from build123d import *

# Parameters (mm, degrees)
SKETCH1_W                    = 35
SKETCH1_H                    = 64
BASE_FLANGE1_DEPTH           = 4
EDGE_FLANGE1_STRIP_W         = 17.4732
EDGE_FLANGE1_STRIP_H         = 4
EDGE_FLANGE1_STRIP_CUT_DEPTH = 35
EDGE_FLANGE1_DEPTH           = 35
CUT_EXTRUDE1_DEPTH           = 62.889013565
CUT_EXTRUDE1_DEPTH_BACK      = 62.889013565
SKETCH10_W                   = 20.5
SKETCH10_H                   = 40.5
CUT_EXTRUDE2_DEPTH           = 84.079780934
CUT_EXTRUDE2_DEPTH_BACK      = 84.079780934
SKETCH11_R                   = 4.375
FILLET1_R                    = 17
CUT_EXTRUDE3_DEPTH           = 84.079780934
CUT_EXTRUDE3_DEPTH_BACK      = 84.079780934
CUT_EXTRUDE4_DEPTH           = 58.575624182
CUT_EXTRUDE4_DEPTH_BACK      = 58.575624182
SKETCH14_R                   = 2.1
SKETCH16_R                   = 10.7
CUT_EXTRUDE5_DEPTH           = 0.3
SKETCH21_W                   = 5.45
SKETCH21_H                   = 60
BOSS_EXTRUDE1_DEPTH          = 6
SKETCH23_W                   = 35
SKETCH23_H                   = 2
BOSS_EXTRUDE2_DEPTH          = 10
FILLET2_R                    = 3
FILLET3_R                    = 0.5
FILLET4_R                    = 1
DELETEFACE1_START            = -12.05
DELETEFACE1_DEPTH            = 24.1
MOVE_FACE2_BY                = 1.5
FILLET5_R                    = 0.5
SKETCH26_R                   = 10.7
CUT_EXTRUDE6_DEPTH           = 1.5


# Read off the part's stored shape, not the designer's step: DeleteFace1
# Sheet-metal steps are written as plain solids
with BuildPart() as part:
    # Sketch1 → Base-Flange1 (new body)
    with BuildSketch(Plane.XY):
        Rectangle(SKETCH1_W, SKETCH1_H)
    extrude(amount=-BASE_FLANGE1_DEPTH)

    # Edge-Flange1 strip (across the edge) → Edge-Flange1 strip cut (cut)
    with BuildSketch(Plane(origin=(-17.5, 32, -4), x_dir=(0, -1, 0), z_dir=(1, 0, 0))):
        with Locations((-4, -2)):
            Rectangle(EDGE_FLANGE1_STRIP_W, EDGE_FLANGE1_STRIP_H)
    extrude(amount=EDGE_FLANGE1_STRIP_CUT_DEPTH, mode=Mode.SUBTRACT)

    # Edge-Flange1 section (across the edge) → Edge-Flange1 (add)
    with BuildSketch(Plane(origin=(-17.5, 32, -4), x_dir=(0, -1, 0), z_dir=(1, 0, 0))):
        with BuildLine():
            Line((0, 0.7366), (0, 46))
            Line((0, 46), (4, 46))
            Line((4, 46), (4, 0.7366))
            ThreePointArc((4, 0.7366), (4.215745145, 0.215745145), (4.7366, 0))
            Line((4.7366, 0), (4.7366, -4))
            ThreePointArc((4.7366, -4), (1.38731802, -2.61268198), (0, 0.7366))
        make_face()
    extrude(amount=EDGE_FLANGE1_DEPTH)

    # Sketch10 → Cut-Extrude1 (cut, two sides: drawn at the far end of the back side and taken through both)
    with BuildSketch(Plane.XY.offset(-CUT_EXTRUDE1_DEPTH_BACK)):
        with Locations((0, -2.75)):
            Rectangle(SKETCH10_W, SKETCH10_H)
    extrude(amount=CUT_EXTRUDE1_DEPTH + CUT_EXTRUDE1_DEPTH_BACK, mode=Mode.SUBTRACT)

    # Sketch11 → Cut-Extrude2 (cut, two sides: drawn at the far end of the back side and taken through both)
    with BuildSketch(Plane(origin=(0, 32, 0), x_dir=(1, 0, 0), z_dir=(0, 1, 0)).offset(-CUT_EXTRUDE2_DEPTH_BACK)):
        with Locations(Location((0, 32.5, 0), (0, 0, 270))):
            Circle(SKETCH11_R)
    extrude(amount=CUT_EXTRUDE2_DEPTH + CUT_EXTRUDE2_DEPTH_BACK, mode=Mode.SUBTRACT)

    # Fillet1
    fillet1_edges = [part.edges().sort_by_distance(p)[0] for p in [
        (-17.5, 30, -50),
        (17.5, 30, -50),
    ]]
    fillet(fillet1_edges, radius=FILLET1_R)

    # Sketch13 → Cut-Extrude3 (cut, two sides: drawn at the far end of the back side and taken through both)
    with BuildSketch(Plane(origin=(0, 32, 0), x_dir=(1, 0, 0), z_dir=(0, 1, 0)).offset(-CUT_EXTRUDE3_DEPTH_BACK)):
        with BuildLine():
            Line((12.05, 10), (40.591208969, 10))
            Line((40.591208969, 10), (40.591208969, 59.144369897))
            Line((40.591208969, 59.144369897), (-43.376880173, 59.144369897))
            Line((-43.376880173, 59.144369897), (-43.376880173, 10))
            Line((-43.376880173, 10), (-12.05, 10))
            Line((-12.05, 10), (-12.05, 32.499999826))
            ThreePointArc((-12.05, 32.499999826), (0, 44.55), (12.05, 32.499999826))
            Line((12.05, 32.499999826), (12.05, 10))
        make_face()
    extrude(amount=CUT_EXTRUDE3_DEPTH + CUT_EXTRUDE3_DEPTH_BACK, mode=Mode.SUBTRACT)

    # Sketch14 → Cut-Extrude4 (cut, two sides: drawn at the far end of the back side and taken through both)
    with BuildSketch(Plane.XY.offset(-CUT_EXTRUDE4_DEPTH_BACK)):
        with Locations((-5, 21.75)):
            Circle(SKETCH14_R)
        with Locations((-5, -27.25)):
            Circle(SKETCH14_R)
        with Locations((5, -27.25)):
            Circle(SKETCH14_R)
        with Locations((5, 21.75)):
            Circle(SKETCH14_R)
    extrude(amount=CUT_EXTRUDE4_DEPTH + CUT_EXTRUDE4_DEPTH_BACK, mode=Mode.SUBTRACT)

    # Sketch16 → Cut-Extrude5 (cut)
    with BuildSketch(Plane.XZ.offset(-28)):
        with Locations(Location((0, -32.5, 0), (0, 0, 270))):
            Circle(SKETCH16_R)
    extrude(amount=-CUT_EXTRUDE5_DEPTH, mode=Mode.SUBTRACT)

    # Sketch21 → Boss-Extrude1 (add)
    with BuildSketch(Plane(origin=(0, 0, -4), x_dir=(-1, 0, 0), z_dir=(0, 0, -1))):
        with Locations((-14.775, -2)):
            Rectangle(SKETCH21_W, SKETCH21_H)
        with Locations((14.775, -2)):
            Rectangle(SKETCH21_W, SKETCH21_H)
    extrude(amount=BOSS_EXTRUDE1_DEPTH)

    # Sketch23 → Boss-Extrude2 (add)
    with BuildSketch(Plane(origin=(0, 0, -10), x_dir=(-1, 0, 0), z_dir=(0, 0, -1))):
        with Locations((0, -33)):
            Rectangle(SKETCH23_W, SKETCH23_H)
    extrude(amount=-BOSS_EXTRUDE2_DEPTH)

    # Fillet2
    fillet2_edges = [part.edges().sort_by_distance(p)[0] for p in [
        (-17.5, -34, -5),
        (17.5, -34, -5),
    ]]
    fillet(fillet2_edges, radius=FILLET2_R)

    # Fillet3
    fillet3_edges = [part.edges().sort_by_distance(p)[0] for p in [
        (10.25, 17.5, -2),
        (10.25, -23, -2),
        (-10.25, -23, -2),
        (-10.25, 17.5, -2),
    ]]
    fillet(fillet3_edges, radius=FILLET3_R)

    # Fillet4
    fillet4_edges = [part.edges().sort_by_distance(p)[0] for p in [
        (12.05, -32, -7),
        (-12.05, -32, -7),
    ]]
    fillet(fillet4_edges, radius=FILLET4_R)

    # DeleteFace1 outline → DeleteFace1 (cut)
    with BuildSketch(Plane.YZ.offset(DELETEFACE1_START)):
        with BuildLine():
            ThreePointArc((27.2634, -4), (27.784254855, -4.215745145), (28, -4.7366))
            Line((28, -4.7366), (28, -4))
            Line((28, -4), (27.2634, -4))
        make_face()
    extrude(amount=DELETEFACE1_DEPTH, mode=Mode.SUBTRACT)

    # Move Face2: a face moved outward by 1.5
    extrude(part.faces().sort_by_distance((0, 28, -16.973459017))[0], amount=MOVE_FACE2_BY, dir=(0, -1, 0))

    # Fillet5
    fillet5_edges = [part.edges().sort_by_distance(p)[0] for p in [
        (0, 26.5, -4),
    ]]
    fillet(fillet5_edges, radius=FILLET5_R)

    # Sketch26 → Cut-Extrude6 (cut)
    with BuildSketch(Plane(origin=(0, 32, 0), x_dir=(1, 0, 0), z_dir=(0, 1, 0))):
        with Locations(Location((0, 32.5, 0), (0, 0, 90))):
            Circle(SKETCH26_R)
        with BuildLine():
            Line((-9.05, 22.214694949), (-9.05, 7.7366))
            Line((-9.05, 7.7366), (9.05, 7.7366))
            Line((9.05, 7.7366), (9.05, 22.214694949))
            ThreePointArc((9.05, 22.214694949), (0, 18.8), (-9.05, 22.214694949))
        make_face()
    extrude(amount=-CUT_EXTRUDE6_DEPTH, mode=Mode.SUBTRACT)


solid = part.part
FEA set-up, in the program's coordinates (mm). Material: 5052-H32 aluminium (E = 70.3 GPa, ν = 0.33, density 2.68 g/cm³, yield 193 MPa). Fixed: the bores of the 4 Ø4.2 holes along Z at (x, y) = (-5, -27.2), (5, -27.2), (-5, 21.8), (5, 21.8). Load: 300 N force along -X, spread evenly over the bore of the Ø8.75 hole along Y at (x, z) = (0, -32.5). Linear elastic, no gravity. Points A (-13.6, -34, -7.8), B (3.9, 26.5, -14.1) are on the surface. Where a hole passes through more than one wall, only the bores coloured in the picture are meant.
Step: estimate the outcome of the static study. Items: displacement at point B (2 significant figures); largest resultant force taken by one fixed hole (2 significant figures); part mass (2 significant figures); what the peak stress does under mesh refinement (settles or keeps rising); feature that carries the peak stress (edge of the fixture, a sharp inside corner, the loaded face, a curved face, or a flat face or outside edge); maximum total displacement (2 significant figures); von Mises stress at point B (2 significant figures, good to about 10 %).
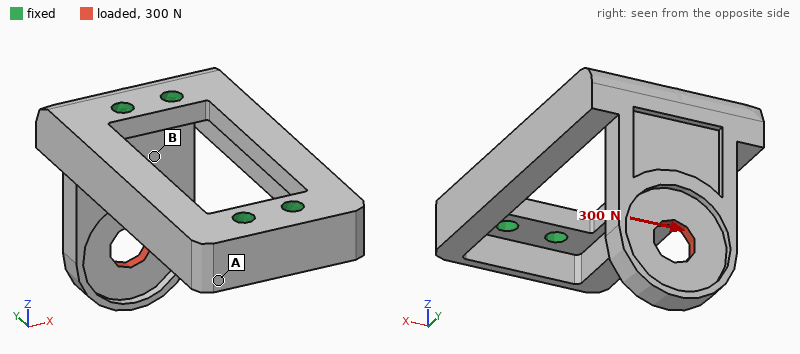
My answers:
14 µm
610 N
36 g
keeps rising
edge of the fixture
52 µm
9.9 MPa
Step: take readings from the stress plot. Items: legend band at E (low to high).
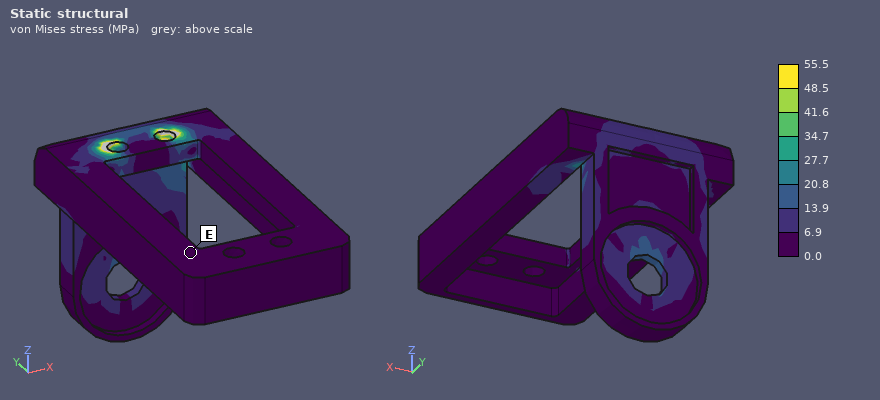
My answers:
0.0 to 6.9 MPa
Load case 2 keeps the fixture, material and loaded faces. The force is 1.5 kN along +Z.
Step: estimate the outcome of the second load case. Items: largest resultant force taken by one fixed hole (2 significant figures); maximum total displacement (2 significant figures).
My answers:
810 N
98 µm
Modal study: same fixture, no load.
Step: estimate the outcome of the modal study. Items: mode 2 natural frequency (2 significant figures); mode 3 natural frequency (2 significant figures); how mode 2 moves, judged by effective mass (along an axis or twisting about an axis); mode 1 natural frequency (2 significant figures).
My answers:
6100 Hz
7900 Hz
along X
3000 Hz
